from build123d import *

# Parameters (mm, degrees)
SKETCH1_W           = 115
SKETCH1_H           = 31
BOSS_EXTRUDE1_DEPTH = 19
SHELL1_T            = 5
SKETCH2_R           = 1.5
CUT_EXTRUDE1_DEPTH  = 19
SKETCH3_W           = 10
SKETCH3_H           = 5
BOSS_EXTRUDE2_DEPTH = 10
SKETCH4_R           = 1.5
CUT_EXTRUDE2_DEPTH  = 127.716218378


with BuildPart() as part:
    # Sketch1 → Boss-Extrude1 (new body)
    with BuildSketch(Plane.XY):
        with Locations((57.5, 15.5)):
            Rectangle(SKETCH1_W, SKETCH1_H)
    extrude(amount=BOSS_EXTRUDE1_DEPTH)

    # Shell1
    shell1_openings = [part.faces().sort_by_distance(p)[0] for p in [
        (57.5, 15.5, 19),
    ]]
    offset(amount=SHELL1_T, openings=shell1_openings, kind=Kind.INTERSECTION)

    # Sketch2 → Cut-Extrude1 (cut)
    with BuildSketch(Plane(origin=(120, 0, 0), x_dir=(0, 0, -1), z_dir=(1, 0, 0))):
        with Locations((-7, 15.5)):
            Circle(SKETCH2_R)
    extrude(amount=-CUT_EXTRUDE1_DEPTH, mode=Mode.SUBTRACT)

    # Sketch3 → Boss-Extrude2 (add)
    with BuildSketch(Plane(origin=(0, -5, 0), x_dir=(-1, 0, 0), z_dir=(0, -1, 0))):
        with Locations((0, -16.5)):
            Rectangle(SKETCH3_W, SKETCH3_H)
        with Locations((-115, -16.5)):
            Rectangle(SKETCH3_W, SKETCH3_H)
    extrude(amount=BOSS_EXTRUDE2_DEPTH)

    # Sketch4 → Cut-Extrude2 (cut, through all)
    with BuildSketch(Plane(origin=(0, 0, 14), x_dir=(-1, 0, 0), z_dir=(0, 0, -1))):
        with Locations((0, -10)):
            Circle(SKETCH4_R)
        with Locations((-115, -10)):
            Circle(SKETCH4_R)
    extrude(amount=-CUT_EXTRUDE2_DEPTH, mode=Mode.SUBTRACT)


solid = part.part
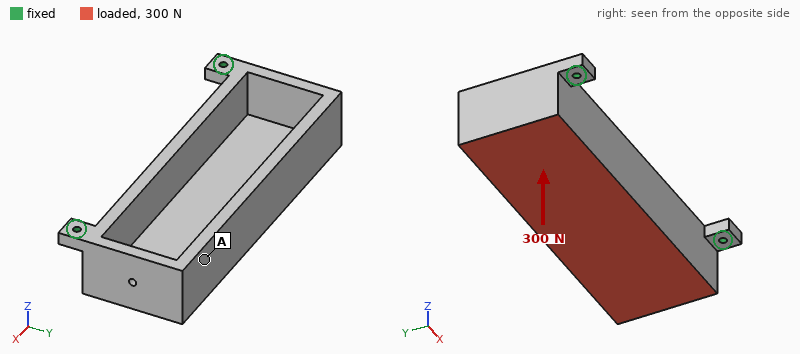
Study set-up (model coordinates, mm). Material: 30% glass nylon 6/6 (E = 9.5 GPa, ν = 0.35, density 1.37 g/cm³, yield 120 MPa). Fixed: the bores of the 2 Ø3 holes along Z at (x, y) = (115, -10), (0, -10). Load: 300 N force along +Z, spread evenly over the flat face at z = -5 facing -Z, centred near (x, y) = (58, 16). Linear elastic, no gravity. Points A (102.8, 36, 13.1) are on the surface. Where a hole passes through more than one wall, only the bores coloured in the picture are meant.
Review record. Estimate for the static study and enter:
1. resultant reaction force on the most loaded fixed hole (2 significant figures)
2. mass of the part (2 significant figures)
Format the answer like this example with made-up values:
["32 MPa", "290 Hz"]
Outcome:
["150 N", "77 g"]
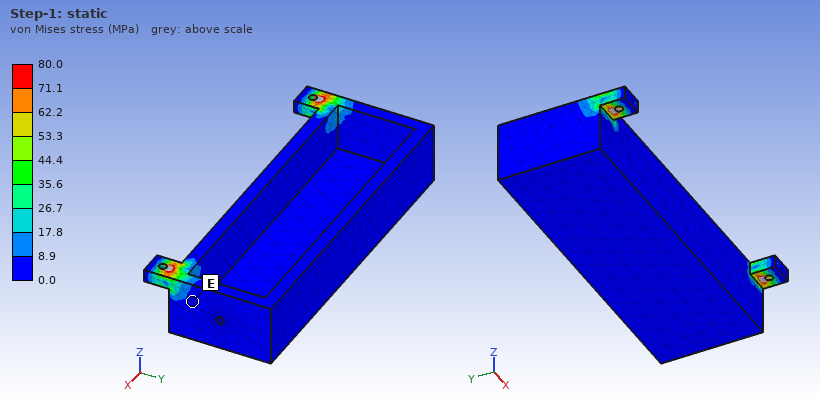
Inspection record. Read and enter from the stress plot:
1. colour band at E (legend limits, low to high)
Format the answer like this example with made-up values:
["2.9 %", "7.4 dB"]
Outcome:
["0.0 to 8.9 MPa"]
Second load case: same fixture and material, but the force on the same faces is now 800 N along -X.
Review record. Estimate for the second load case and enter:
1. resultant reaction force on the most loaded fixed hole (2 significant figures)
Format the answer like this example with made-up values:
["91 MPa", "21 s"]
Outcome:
["450 N"]
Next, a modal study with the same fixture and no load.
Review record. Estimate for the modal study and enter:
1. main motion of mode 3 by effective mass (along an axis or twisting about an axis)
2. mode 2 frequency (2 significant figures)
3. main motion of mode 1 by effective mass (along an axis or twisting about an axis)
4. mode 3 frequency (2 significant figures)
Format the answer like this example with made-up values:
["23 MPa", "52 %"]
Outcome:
["along Y", "760 Hz", "along Z", "1700 Hz"]
